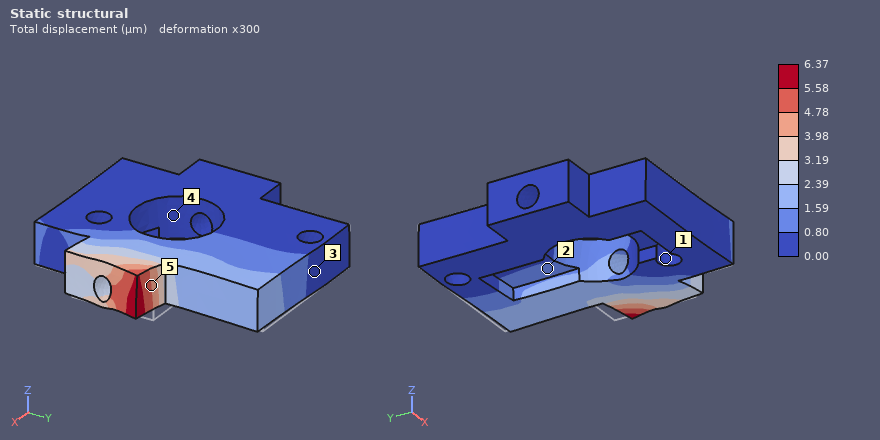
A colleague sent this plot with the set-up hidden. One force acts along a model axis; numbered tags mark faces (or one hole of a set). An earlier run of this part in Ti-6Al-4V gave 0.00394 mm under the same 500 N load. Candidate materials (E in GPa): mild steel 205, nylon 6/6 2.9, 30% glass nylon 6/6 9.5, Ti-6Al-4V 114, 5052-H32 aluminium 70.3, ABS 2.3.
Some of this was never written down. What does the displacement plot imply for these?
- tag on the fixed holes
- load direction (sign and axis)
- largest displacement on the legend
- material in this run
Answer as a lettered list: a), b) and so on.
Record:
a) 1
b) -Y
c) 6.37 µm
d) 5052-H32 aluminium
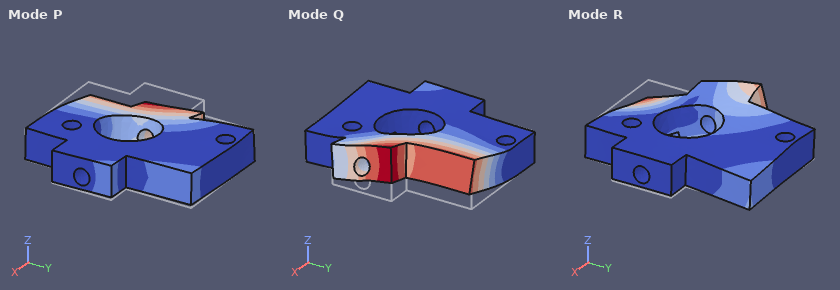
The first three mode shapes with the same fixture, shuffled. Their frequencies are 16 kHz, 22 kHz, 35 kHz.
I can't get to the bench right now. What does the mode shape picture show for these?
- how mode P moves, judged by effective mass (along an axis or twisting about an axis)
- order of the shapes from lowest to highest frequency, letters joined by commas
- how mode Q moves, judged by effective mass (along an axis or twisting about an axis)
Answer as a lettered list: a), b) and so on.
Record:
a) along Z
b) P, Q, R
c) along Z
